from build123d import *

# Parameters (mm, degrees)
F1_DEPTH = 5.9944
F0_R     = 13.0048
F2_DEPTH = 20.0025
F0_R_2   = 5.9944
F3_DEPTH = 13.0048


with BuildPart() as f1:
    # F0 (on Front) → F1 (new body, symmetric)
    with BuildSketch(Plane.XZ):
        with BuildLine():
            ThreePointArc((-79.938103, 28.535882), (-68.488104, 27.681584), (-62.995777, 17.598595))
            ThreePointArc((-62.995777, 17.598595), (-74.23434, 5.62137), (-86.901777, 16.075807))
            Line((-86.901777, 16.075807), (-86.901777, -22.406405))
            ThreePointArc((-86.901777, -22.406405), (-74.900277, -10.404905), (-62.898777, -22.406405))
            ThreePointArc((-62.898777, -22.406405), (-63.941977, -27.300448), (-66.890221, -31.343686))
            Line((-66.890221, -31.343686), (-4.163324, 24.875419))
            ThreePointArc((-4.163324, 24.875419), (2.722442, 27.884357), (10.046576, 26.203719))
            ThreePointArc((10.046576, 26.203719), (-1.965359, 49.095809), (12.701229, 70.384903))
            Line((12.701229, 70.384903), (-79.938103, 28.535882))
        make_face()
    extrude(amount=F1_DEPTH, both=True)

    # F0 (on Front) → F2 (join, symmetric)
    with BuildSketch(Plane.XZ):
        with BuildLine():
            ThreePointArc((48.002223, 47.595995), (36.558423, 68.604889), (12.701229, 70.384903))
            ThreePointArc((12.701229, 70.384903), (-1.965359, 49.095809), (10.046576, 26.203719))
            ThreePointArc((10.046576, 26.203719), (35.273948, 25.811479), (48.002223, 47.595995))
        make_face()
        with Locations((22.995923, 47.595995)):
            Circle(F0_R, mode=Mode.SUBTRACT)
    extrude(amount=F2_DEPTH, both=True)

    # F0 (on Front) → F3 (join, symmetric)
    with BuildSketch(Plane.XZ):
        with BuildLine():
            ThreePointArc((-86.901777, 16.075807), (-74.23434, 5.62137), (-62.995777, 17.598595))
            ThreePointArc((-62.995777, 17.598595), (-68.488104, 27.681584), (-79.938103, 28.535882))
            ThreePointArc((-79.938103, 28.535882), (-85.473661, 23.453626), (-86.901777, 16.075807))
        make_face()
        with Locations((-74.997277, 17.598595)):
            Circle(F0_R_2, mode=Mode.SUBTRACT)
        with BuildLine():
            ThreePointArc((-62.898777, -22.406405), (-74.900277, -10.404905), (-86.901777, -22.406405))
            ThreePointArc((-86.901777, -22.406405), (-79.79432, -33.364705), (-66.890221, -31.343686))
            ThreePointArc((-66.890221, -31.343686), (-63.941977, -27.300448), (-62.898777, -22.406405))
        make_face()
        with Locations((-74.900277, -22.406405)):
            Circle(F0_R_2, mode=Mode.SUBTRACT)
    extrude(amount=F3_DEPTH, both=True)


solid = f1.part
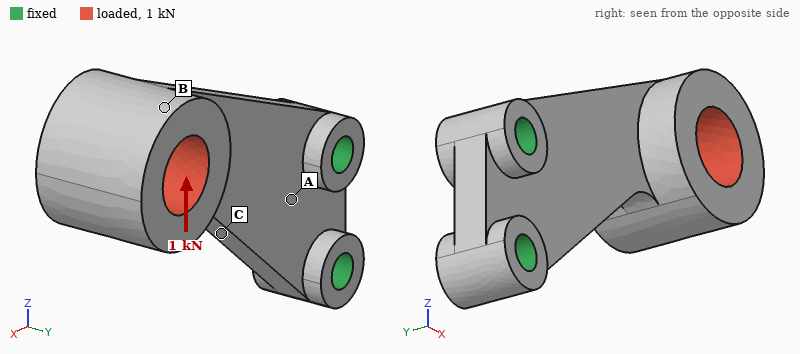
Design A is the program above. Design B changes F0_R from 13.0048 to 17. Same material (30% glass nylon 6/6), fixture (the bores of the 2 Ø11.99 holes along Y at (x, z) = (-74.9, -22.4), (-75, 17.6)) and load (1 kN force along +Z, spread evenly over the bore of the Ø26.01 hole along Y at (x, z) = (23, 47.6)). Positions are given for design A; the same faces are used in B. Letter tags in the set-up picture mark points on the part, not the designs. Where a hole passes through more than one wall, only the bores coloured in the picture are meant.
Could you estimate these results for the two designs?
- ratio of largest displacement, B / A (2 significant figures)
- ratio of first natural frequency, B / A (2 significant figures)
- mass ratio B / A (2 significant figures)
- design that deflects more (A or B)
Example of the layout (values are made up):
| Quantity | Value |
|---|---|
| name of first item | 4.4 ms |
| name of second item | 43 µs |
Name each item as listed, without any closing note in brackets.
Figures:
| Quantity | Value |
|---|---|
| ratio of largest displacement, B / A | 1.1 |
| ratio of first natural frequency, B / A | 1.1 |
| mass ratio B / A | 0.87 |
| design that deflects more | B |
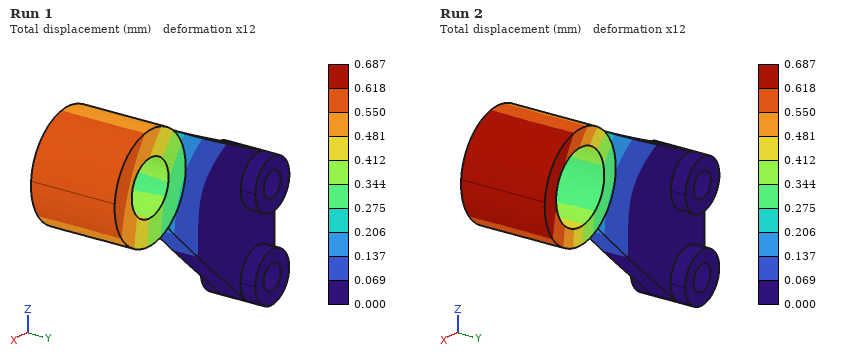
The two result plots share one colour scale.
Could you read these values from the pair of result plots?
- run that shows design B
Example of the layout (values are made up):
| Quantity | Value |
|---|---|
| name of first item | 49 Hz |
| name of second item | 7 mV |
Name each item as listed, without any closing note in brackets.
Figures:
| Quantity | Value |
|---|---|
| run that shows design B | Run 2 |
